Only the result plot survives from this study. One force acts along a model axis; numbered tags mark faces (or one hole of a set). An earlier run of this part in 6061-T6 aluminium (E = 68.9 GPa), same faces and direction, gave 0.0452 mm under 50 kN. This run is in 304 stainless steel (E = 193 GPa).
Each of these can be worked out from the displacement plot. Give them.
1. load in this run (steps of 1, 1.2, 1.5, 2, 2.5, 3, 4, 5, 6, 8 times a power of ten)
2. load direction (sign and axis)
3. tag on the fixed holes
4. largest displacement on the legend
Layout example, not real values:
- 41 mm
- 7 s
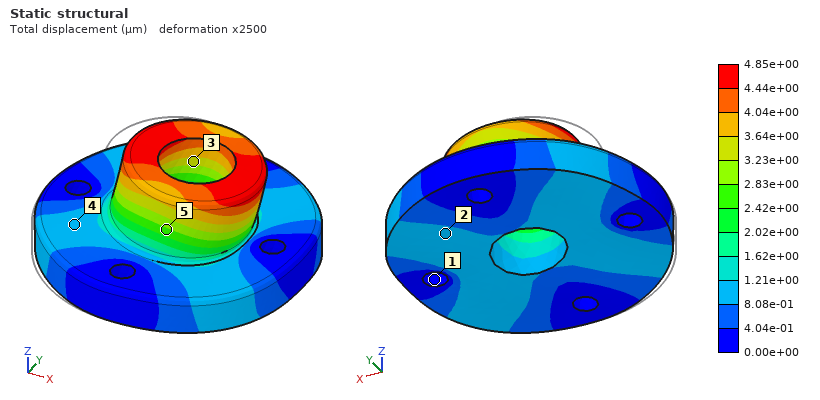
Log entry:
- 15 kN
- +X
- 1
- 4.85e+00 µm
